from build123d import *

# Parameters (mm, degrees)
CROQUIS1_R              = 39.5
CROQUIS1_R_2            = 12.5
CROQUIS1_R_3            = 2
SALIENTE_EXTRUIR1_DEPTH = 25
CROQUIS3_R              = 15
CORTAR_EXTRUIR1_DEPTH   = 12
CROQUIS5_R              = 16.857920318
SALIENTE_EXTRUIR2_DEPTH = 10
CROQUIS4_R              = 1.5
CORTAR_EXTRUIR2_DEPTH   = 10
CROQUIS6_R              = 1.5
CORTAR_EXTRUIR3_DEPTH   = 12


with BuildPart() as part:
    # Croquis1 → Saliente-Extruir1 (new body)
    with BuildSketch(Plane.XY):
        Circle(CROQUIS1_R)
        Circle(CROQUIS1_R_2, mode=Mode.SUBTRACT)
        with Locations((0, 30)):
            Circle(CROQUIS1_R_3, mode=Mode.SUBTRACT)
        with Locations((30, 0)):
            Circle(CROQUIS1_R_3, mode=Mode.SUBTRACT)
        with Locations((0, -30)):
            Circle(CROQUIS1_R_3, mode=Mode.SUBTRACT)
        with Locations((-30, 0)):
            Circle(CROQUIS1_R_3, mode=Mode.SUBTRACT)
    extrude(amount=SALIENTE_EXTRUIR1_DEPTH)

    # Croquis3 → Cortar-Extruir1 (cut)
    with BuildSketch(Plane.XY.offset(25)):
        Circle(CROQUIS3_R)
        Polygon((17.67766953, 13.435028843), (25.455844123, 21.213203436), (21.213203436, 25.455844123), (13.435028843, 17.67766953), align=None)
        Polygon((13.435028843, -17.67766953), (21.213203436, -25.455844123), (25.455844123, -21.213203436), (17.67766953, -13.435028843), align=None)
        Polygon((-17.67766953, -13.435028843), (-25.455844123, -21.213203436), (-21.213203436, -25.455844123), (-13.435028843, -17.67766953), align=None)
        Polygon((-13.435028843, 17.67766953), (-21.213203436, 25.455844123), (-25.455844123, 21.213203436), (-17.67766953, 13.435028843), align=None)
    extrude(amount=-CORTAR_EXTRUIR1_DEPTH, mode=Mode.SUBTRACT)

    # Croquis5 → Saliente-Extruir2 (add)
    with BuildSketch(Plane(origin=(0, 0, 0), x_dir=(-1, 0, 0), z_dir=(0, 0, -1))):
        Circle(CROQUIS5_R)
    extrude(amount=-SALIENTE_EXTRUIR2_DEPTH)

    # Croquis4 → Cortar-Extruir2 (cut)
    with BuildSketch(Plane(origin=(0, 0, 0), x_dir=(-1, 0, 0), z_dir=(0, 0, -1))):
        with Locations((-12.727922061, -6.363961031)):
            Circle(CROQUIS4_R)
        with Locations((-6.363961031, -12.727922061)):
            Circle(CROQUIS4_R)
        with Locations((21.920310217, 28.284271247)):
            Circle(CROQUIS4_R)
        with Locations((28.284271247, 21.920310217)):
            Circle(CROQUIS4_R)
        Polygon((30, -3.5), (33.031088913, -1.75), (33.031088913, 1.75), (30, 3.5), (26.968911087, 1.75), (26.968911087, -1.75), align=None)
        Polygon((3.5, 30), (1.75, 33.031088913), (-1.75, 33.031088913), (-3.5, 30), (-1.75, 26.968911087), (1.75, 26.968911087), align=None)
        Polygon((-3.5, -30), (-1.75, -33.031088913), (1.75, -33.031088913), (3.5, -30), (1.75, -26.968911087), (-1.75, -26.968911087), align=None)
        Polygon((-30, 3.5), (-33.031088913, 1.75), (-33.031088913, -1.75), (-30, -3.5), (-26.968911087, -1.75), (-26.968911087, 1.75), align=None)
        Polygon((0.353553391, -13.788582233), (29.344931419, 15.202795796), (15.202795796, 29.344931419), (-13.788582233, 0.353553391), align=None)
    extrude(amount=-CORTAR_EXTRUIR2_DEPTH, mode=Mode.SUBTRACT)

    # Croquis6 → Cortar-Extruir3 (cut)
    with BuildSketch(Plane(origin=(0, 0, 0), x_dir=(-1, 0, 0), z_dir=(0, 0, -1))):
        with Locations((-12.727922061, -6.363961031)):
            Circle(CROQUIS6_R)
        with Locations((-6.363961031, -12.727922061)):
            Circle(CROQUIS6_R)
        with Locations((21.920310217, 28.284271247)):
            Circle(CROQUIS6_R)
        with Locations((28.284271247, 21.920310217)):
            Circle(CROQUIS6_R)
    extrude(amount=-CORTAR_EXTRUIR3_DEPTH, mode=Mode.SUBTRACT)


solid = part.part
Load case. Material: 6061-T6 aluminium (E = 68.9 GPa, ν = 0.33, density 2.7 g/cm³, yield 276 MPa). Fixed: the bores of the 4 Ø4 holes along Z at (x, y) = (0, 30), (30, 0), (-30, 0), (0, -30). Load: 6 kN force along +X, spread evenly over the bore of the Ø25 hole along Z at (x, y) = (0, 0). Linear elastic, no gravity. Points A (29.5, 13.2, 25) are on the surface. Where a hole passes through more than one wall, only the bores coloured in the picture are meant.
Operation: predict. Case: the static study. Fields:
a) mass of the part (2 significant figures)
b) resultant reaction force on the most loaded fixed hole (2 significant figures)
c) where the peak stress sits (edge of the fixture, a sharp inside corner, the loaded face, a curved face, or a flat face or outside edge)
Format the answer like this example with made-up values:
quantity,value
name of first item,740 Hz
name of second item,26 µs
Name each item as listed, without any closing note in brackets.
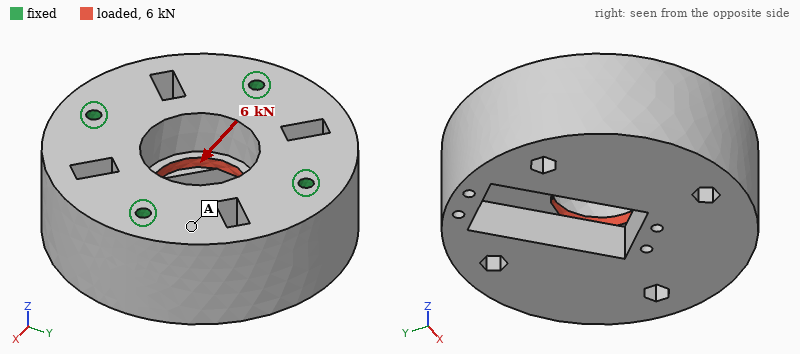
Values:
quantity,value
mass of the part,270 g
resultant reaction force on the most loaded fixed hole,1.8 kN
where the peak stress sits,a curved face
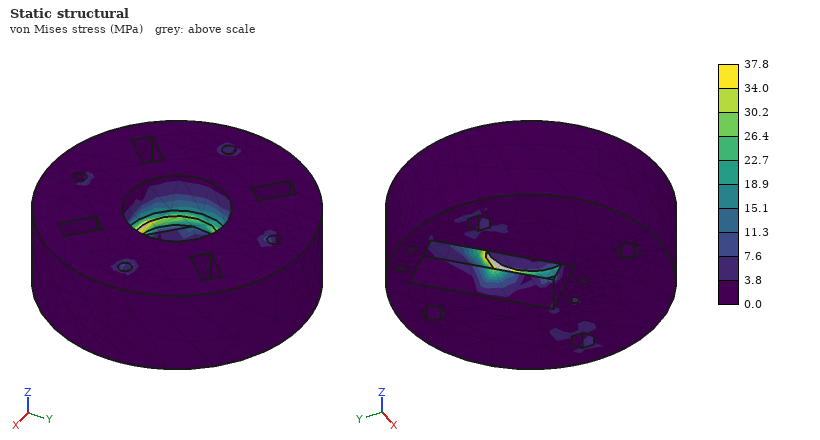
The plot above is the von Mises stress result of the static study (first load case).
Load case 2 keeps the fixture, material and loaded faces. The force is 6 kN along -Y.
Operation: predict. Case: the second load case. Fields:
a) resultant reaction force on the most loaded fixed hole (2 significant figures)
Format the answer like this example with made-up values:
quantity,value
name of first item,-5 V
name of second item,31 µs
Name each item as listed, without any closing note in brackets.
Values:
quantity,value
resultant reaction force on the most loaded fixed hole,1.8 kN
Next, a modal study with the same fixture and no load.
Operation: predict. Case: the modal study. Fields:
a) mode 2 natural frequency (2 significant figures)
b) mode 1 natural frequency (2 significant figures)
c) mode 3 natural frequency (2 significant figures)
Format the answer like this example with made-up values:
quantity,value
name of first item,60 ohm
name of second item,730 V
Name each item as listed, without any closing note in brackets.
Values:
quantity,value
mode 2 natural frequency,18 kHz
mode 1 natural frequency,16 kHz
mode 3 natural frequency,18 kHz
